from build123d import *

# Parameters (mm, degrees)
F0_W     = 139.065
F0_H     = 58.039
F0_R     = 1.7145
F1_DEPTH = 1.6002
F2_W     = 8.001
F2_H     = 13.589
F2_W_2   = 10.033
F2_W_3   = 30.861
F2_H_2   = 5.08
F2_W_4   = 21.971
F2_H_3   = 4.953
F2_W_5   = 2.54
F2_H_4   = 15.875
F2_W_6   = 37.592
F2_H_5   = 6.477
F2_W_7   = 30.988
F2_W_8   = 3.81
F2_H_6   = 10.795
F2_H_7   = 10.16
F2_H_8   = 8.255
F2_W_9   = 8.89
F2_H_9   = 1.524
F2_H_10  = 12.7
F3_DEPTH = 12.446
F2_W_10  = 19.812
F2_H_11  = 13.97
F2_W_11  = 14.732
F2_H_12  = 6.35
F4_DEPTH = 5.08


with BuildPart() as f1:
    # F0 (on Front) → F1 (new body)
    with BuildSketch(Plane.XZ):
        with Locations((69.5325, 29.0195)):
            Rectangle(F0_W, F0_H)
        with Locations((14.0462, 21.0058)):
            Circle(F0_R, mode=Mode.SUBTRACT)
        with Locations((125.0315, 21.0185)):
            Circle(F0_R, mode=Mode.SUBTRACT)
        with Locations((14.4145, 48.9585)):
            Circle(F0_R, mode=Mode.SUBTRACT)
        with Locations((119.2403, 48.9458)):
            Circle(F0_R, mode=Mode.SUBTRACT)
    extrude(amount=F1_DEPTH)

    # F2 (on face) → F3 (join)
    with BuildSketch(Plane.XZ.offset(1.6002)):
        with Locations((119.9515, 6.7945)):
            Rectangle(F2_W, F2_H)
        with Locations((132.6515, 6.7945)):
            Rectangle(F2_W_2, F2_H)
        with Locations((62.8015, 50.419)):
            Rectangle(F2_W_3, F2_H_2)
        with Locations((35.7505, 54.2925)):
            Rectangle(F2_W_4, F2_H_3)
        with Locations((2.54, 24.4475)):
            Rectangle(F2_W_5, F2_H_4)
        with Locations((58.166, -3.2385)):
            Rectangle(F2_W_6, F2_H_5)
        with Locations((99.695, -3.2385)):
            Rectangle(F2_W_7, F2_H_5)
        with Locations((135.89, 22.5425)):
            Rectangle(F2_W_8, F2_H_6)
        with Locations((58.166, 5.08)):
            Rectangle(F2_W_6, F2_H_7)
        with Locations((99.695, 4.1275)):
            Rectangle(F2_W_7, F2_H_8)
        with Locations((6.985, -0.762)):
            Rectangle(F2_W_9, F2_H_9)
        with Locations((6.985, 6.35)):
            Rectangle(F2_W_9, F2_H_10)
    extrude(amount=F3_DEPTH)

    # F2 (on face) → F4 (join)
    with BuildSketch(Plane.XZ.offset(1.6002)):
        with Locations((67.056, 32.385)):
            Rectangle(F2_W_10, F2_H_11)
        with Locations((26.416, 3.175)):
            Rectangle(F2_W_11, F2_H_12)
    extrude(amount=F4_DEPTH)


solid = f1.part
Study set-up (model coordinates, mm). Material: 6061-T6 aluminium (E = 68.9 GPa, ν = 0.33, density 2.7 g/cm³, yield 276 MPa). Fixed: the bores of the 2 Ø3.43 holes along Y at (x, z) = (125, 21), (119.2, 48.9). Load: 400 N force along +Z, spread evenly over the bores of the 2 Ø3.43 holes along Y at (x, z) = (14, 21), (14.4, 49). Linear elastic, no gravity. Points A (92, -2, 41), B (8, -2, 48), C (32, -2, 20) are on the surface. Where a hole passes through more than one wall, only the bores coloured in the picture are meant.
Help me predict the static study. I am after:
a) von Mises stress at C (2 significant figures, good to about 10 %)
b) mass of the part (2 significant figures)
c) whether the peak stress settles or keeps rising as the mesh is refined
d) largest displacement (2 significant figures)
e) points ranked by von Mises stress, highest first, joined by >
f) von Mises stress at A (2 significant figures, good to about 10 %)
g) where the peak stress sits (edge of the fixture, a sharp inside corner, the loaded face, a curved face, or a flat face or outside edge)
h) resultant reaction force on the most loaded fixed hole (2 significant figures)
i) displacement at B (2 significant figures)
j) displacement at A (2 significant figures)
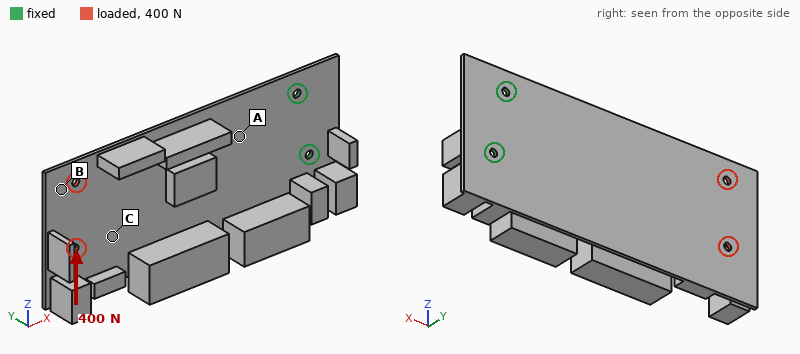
10 MPa
100 g
keeps rising
0.23 mm
A > C > B
20 MPa
edge of the fixture
1.5 kN
0.21 mm
0.035 mm
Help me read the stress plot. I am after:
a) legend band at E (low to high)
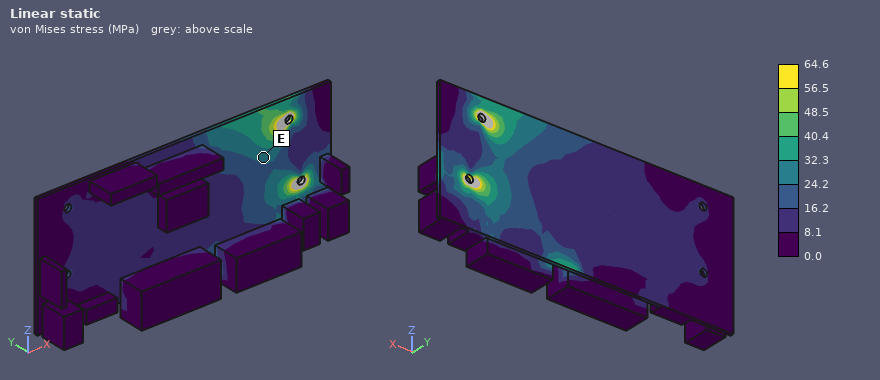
24.2 to 32.3 MPa
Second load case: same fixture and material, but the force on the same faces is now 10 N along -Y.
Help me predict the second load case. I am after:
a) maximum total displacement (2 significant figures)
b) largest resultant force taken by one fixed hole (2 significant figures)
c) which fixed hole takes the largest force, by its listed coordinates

1.7 mm
11 N
(119.2, 48.9)
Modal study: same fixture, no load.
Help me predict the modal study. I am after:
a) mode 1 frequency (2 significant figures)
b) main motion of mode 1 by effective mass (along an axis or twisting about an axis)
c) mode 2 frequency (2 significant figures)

77 Hz
along Y
290 Hz
